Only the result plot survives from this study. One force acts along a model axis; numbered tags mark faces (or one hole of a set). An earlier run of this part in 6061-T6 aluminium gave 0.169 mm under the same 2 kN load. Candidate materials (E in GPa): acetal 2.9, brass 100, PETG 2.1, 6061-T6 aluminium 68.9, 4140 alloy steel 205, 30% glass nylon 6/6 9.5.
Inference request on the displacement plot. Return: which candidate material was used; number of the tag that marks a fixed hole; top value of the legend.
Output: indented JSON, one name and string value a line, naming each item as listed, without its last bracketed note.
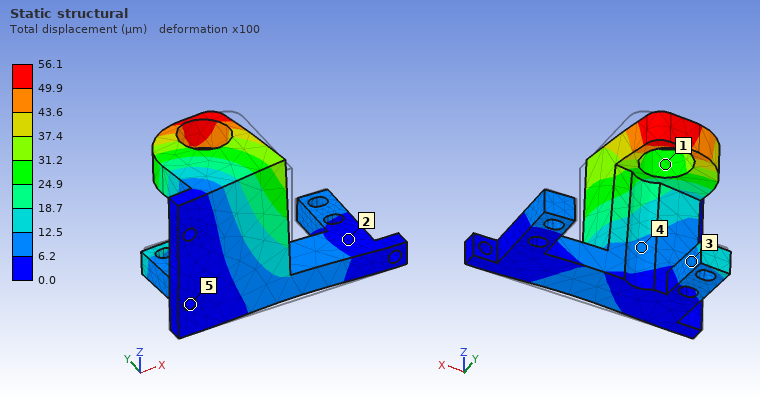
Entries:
{
  "which candidate material was used": "4140 alloy steel",
  "number of the tag that marks a fixed hole": "5",
  "top value of the legend": "56.1 µm"
}
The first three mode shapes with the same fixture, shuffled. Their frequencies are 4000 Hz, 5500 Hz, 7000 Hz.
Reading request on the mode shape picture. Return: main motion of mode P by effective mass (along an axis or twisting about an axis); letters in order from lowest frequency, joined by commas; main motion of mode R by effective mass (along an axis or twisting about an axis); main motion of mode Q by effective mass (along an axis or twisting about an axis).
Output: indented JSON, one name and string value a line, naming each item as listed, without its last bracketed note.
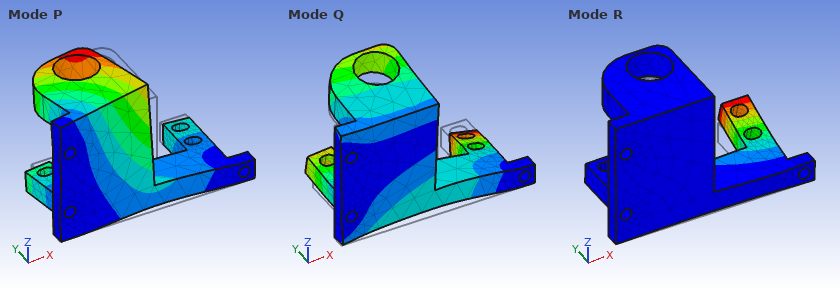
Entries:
{
  "main motion of mode P by effective mass": "along Y",
  "letters in order from lowest frequency, joined by commas": "P, R, Q",
  "main motion of mode R by effective mass": "along Z",
  "main motion of mode Q by effective mass": "along Z"
}
